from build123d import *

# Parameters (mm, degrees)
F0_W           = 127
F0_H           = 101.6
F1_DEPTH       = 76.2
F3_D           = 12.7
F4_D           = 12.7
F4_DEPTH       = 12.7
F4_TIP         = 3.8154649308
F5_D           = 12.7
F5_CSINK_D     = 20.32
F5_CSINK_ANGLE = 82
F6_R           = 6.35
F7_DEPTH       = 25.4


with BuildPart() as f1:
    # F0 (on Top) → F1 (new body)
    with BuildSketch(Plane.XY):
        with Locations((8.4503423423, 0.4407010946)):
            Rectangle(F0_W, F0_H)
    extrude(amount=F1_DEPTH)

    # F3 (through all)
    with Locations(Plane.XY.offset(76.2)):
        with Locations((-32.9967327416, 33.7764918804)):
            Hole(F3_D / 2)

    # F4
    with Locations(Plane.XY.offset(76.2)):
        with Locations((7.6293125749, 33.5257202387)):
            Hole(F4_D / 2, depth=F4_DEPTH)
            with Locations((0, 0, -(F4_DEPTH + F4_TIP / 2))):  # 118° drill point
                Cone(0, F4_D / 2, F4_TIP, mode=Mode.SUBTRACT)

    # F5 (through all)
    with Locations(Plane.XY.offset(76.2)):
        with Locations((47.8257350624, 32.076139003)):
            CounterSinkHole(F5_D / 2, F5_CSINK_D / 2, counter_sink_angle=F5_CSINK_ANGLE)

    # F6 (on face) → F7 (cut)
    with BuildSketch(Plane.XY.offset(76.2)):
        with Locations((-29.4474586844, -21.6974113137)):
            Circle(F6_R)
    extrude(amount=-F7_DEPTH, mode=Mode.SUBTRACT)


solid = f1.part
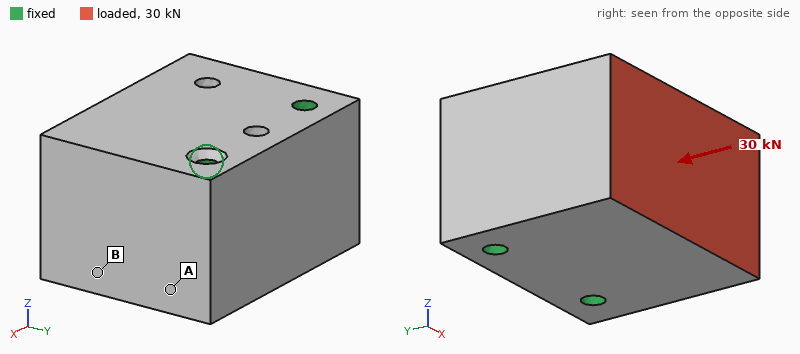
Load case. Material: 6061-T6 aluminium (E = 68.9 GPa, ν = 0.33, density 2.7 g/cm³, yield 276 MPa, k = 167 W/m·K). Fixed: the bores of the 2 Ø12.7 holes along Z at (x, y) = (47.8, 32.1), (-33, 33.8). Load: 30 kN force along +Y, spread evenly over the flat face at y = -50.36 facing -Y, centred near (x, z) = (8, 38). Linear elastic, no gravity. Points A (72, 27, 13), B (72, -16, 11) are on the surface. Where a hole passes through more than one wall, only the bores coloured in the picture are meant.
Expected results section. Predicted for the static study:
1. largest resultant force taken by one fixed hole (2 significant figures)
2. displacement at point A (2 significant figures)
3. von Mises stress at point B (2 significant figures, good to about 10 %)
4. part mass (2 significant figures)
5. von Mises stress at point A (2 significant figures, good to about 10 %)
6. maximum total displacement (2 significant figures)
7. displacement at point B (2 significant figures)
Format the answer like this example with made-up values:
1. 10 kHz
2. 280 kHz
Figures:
1. 15 kN
2. 1.4 µm
3. 3.0 MPa
4. 2.6 kg
5. 1.5 MPa
6. 5.1 µm
7. 2.9 µm
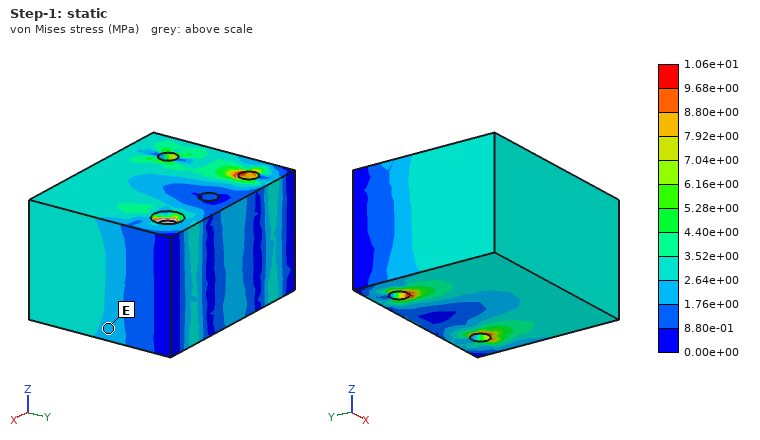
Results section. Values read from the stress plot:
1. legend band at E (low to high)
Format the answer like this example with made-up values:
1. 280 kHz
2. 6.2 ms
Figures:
1. 1.76e+00 to 2.64e+00 MPa
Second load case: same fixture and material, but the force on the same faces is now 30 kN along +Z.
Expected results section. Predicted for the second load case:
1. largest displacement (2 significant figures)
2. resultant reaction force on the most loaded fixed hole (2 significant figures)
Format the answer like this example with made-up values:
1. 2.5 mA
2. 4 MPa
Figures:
1. 45 µm
2. 15 kN
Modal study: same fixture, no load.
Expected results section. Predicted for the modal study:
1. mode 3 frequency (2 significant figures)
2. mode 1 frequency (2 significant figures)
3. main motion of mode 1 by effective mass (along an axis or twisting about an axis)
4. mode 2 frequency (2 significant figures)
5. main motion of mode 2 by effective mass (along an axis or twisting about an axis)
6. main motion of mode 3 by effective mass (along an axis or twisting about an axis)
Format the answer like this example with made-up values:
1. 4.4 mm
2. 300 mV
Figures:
1. 8000 Hz
2. 5100 Hz
3. along Z
4. 6600 Hz
5. along X
6. twisting about Y
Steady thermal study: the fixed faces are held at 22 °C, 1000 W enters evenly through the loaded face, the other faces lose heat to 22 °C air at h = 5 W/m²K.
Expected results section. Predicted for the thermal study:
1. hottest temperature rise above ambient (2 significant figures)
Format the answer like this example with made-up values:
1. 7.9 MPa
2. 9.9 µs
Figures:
1. 56 K
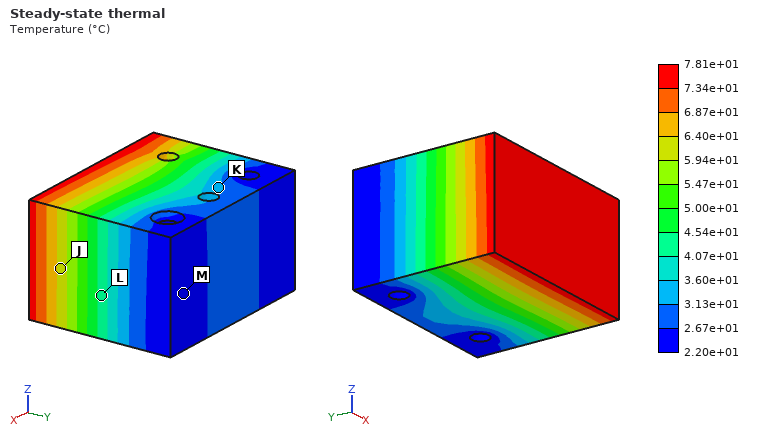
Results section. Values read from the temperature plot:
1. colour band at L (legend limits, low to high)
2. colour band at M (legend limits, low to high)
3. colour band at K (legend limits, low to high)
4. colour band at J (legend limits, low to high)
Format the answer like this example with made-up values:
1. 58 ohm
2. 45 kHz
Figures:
1. 4.07e+01 to 4.54e+01 °C
2. 2.20e+01 to 2.67e+01 °C
3. 3.13e+01 to 3.60e+01 °C
4. 5.94e+01 to 6.40e+01 °C
